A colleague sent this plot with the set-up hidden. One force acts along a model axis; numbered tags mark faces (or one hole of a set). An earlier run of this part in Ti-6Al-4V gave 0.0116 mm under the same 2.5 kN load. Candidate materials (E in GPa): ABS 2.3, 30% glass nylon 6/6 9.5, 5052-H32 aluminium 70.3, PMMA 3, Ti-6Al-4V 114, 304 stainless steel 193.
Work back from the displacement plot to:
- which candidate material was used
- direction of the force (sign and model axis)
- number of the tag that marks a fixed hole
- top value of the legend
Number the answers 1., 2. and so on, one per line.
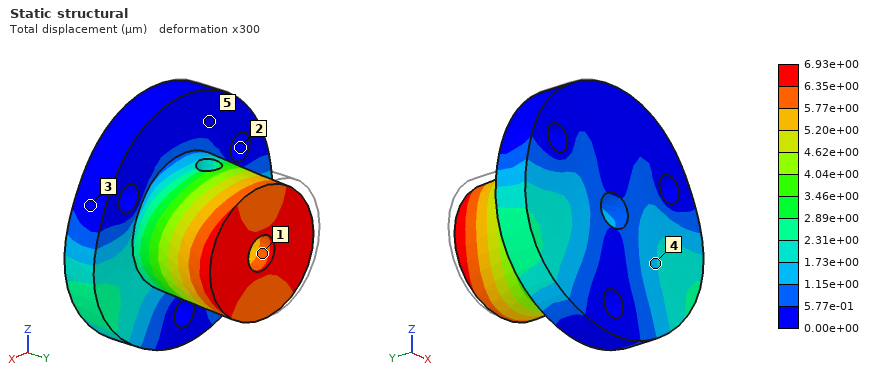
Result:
1. 304 stainless steel
2. +X
3. 2
4. 6.93e+00 µm
